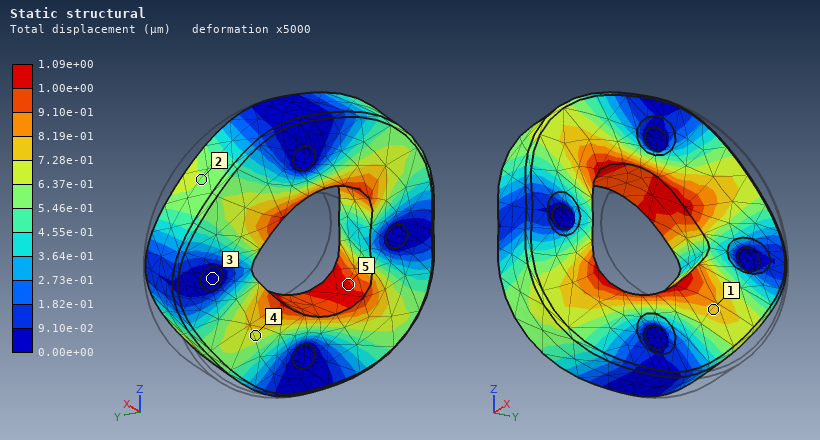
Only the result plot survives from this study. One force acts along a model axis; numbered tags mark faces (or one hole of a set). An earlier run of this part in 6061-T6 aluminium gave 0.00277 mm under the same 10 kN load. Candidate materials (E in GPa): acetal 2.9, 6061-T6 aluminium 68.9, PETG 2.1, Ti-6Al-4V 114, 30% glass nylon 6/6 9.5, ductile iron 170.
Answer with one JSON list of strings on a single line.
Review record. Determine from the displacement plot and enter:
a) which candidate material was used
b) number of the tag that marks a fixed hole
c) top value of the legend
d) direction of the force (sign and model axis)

["ductile iron", "3", "1.09e+00 µm", "-Y"]
